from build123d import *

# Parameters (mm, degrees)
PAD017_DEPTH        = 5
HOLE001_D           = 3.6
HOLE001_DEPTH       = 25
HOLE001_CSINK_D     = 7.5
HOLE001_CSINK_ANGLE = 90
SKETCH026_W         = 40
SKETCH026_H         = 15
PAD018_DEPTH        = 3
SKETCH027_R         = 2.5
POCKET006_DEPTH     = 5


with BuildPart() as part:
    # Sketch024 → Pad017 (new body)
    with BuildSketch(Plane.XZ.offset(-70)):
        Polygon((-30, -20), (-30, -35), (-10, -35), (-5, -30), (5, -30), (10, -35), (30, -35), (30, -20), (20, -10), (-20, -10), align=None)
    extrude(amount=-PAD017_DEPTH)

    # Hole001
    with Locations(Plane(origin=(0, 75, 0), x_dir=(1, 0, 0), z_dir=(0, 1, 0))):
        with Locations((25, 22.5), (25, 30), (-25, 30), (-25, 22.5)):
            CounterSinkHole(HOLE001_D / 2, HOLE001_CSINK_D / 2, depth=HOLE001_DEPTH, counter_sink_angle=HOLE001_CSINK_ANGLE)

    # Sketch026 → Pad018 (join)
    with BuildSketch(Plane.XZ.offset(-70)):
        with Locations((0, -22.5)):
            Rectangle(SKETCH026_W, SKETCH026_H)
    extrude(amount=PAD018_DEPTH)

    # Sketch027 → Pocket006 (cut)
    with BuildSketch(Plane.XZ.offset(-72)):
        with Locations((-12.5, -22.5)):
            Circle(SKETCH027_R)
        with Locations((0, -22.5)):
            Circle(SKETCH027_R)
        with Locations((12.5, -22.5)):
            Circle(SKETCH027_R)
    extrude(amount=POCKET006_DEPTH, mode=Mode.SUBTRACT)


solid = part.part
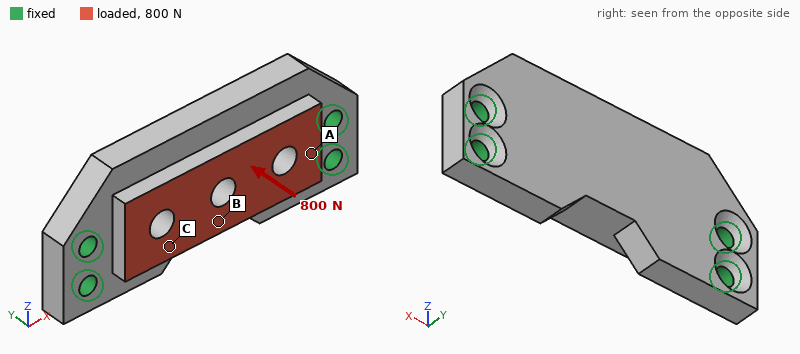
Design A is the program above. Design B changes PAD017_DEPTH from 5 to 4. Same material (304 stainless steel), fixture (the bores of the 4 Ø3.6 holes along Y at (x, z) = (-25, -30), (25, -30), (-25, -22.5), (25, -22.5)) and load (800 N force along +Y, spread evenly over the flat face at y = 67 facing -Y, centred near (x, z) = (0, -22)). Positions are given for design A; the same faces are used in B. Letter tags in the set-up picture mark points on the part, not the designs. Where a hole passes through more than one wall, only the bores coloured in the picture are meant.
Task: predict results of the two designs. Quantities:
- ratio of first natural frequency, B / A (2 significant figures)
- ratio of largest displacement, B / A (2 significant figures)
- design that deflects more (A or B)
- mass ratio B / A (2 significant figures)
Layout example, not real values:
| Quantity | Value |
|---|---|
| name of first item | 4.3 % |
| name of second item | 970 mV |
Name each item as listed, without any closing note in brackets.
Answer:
| Quantity | Value |
|---|---|
| ratio of first natural frequency, B / A | 0.96 |
| ratio of largest displacement, B / A | 1.3 |
| design that deflects more | B |
| mass ratio B / A | 0.85 |
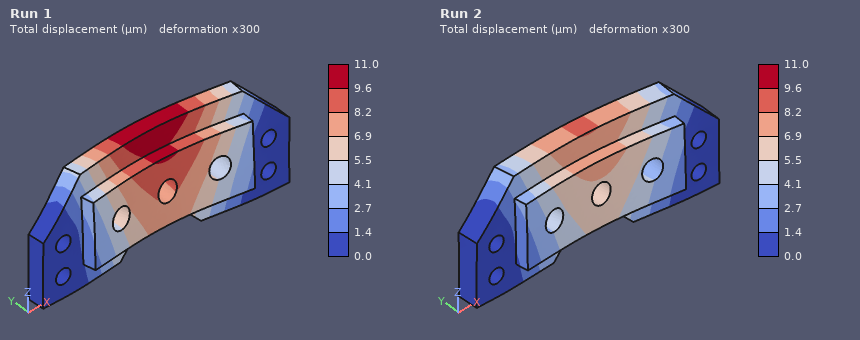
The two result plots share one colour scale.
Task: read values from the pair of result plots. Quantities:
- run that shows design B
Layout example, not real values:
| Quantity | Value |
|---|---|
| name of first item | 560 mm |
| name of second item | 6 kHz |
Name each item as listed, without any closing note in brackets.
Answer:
| Quantity | Value |
|---|---|
| run that shows design B | Run 1 |
